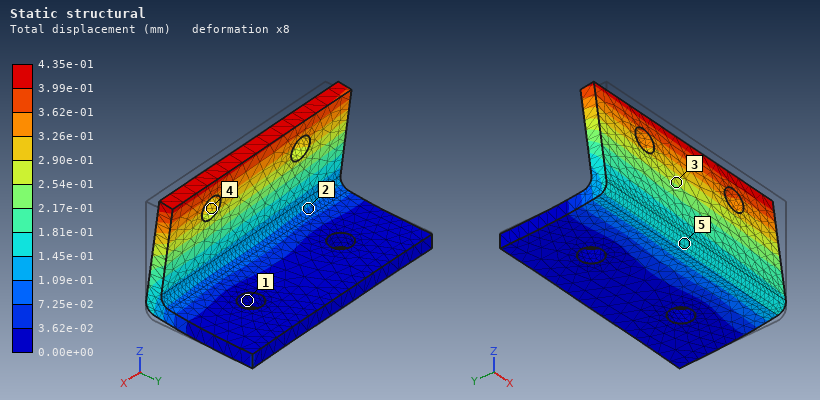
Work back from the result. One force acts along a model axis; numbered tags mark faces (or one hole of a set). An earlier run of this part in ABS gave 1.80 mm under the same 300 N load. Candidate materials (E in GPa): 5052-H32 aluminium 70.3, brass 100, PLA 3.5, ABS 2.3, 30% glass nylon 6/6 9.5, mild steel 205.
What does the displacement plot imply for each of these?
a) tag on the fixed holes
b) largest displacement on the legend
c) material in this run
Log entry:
1
4.35e-01 mm
30% glass nylon 6/6
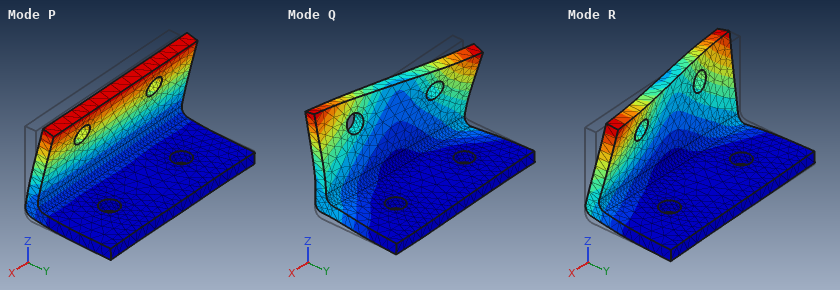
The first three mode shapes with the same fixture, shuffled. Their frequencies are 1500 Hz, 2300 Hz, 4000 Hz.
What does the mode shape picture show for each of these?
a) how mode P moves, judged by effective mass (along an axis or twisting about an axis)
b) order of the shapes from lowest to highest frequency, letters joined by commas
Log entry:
along Y
P, R, Q
